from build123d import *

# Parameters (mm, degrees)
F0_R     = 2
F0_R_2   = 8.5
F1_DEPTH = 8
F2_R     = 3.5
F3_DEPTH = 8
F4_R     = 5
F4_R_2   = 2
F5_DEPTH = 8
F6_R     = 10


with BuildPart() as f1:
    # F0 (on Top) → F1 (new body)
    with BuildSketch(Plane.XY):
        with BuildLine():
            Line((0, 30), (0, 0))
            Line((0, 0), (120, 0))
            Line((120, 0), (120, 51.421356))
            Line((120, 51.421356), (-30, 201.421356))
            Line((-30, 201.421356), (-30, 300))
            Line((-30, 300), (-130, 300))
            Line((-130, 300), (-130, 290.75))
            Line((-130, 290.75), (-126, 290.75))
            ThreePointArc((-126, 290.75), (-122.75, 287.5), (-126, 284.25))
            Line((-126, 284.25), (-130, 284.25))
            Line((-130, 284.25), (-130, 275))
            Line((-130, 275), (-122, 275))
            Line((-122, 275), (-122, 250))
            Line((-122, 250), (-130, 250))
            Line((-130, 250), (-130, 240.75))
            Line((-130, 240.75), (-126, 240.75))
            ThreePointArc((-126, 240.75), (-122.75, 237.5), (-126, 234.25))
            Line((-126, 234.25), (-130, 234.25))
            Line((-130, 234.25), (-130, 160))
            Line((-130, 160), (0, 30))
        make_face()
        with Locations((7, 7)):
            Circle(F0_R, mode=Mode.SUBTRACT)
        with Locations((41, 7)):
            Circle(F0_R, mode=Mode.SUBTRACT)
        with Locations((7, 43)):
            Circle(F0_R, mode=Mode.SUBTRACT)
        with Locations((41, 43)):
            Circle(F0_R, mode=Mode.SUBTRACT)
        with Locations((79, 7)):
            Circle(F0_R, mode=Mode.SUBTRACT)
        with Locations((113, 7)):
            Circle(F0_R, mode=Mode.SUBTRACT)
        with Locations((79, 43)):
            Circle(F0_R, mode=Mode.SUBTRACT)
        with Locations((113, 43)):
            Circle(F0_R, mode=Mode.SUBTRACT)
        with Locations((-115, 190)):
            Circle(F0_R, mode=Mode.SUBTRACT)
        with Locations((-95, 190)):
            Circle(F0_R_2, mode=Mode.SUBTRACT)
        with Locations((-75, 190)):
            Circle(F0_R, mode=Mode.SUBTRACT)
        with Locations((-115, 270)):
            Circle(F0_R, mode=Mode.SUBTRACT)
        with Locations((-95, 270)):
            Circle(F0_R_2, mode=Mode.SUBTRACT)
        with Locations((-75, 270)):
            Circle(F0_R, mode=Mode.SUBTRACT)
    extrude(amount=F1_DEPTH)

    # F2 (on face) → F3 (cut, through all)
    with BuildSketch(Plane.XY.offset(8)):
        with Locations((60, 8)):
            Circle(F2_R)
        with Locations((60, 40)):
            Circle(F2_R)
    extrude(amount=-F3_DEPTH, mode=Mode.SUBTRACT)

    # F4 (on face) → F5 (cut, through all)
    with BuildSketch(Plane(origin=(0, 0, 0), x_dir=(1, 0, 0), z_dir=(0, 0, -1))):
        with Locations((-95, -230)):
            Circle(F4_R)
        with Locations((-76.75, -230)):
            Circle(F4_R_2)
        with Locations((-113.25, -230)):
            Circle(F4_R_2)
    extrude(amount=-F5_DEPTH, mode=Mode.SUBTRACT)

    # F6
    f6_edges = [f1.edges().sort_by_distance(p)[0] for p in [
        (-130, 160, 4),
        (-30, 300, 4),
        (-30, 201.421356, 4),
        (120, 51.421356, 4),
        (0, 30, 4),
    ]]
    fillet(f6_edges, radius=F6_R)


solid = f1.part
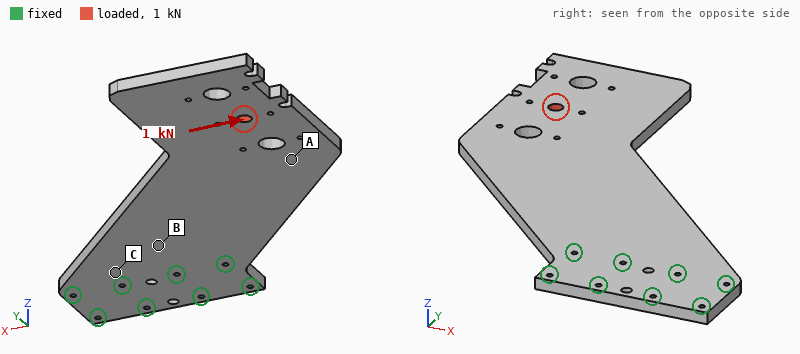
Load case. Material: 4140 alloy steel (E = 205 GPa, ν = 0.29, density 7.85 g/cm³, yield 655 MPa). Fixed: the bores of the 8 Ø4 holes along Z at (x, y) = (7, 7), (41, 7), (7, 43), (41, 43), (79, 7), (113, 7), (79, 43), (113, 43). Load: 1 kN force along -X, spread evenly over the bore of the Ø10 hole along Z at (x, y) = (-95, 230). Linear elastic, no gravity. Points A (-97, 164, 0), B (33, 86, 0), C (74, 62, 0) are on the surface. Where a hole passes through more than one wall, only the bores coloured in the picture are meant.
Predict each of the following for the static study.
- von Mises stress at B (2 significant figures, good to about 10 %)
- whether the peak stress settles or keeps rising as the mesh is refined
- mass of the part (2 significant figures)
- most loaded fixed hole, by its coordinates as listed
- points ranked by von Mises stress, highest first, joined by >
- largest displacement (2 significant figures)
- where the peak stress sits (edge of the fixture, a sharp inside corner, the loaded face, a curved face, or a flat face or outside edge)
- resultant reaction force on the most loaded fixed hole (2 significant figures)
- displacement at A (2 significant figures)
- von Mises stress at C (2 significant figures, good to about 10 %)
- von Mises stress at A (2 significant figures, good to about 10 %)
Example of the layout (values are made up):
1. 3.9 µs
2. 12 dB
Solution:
1. 5.0 MPa
2. keeps rising
3. 2.2 kg
4. (7, 43)
5. C > B > A
6. 42 µm
7. edge of the fixture
8. 1.9 kN
9. 20 µm
10. 7.0 MPa
11. 1.7 MPa
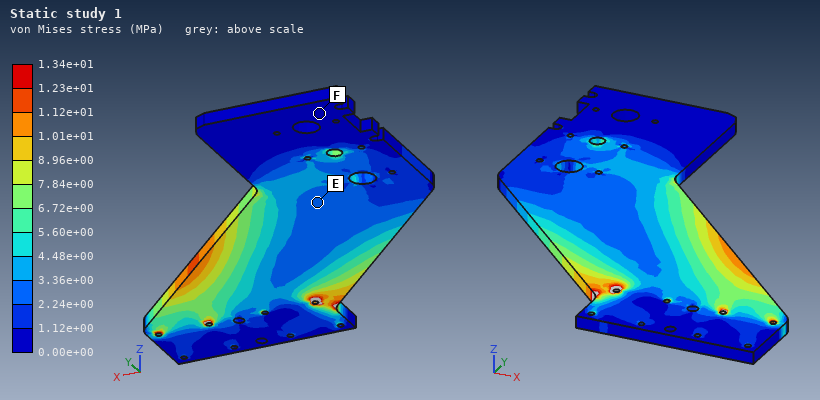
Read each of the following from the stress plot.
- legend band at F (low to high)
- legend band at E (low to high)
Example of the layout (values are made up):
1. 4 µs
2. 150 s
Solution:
1. 0.00e+00 to 1.12e+00 MPa
2. 2.24e+00 to 3.36e+00 MPa
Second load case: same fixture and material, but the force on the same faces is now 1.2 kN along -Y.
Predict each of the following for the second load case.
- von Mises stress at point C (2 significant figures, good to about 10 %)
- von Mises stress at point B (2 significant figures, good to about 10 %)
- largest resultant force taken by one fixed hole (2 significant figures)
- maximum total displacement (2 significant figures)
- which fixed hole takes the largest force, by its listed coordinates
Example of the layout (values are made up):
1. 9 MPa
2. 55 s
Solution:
1. 4.8 MPa
2. 2.9 MPa
3. 2.1 kN
4. 36 µm
5. (7, 43)
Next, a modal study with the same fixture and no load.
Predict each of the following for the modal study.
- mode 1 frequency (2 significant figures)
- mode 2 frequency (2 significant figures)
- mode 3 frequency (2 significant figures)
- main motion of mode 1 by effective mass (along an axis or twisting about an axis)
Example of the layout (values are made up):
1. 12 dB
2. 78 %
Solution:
1. 84 Hz
2. 380 Hz
3. 560 Hz
4. along Z
